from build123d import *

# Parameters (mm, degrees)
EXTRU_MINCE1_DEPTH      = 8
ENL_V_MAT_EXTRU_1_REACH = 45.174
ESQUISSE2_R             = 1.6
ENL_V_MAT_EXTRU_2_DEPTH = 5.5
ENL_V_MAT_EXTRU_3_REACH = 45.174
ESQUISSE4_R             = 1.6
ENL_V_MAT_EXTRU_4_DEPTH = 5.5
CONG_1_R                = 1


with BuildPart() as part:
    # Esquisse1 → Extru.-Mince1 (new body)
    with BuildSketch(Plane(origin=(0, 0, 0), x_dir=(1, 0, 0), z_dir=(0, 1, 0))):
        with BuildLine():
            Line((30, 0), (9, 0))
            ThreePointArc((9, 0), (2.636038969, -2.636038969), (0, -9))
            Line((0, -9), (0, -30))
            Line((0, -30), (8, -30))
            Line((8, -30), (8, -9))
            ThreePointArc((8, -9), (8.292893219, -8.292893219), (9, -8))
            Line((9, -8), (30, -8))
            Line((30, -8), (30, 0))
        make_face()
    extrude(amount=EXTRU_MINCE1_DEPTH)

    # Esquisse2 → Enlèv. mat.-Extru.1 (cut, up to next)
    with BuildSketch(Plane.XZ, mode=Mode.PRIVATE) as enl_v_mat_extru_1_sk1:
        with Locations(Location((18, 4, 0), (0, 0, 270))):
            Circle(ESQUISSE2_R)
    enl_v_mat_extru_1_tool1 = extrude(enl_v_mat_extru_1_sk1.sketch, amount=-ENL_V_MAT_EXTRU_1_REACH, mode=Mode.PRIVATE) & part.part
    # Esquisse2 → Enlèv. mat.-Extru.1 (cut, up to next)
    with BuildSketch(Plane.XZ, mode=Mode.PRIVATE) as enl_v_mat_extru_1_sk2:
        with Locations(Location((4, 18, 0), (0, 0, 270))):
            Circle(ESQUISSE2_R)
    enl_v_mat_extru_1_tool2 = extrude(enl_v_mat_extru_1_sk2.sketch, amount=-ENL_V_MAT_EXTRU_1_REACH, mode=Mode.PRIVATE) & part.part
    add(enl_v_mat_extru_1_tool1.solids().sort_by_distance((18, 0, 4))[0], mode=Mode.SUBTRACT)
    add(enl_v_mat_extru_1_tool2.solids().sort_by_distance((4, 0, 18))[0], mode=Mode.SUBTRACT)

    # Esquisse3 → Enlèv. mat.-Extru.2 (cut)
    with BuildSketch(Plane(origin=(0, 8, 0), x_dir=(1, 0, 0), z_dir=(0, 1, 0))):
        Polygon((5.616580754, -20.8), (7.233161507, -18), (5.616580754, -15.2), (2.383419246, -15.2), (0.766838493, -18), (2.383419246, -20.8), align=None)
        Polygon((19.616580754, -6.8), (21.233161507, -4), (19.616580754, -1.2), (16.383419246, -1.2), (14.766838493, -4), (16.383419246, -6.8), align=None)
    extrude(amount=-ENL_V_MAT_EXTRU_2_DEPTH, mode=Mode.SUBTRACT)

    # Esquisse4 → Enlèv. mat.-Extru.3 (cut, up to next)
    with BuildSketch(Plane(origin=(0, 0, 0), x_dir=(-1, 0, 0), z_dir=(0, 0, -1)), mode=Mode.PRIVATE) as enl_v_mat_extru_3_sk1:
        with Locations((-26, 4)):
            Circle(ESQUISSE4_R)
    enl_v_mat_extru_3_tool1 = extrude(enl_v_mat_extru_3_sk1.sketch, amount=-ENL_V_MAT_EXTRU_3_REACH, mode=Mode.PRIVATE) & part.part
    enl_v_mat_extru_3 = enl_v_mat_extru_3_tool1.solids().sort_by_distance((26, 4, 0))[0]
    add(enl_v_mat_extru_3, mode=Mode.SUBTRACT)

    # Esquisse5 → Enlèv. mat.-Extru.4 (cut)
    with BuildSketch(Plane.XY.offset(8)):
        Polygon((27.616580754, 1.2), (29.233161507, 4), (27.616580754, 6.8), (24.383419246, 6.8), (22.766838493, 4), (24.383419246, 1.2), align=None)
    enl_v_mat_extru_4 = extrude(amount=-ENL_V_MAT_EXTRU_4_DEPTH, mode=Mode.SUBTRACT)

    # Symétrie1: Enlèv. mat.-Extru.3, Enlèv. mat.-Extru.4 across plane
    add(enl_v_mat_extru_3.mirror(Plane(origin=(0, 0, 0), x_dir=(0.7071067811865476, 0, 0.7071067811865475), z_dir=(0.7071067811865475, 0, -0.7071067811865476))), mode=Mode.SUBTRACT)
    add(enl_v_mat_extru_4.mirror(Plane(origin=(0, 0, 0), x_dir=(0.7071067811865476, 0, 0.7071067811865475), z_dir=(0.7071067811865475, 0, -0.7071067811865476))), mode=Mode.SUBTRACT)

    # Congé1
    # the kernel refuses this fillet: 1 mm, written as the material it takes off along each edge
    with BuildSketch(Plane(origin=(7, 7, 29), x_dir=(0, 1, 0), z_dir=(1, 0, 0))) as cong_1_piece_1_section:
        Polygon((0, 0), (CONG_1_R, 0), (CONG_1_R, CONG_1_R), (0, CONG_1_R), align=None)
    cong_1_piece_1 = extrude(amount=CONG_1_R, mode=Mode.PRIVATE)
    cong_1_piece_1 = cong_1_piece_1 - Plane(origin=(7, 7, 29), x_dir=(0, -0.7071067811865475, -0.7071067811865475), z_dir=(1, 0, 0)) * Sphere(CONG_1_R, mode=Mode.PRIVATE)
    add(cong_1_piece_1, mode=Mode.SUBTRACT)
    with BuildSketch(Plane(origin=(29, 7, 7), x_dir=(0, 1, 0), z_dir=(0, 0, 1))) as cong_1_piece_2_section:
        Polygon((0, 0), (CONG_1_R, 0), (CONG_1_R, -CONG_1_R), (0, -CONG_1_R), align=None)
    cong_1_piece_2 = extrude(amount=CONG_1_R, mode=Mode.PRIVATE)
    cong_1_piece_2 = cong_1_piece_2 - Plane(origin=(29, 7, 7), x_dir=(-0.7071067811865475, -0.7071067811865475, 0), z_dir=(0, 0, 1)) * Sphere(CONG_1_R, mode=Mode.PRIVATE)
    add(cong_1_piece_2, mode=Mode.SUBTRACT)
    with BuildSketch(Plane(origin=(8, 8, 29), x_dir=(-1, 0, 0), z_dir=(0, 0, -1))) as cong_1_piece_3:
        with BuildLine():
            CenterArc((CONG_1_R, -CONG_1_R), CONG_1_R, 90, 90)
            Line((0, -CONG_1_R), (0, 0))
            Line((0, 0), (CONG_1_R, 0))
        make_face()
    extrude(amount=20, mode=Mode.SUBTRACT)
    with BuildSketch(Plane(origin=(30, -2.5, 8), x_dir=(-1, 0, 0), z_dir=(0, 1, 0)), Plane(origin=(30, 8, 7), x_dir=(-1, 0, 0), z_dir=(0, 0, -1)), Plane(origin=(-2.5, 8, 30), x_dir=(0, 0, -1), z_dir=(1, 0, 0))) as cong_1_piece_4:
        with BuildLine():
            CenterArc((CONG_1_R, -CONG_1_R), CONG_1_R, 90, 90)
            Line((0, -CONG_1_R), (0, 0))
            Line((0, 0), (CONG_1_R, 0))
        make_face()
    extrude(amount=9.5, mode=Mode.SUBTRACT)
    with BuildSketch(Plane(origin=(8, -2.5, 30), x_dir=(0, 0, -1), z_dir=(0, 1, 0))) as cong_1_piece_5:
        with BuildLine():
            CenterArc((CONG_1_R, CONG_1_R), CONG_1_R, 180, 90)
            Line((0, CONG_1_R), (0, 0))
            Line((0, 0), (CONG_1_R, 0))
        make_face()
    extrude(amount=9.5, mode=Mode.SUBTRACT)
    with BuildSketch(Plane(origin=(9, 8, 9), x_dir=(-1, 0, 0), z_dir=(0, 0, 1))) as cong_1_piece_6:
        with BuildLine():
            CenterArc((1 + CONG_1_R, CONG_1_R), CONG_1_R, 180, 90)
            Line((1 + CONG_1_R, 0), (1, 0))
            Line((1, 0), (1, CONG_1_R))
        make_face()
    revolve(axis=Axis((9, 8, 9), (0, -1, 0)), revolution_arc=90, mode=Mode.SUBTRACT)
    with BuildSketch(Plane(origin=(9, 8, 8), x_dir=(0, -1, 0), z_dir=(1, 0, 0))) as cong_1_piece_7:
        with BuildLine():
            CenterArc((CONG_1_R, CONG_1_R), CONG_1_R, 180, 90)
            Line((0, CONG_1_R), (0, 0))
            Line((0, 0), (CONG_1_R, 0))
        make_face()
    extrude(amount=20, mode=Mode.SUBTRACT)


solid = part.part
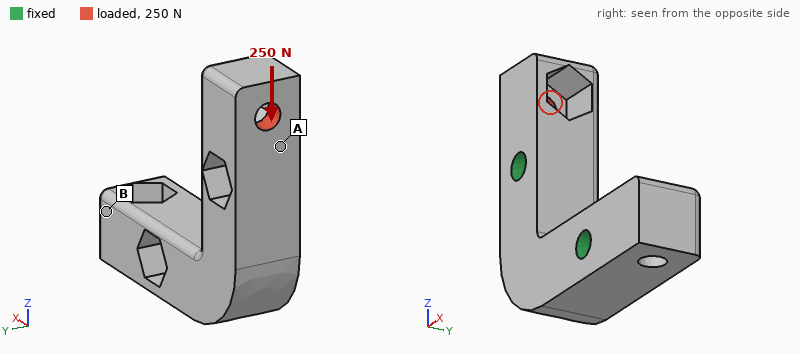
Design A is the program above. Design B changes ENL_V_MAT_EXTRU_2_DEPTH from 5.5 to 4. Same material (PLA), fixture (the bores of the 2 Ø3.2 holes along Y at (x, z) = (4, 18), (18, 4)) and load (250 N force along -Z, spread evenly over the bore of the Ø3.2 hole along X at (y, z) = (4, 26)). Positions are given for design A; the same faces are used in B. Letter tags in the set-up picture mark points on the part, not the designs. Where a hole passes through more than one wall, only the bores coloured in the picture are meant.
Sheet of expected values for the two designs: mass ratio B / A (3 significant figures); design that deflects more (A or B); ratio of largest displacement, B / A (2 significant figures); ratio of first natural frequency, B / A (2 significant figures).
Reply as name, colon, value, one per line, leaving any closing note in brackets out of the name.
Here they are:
mass ratio B / A: 1.02
design that deflects more: A
ratio of largest displacement, B / A: 0.68
ratio of first natural frequency, B / A: 1.4
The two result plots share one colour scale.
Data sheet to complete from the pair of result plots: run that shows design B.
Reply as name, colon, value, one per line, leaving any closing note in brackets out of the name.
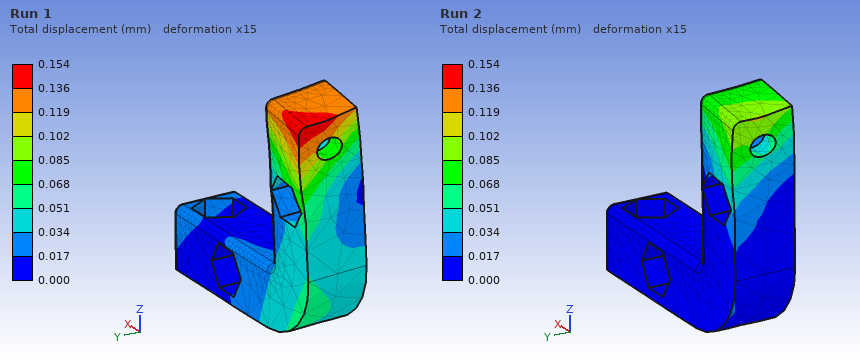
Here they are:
run that shows design B: Run 2
